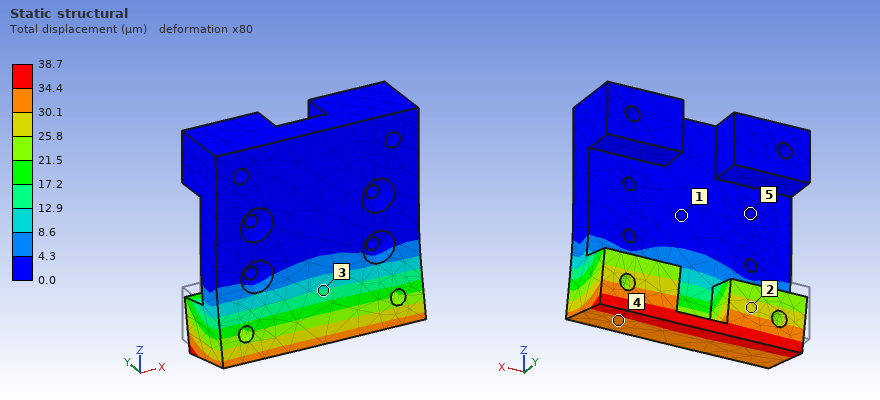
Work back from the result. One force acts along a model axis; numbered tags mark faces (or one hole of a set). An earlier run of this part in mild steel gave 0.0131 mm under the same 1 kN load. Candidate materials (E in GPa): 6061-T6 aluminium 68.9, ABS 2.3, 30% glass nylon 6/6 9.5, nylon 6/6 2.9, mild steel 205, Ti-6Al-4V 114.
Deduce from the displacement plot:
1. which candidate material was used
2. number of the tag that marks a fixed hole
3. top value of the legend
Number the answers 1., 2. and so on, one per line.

1. 6061-T6 aluminium
2. 5
3. 38.7 µm
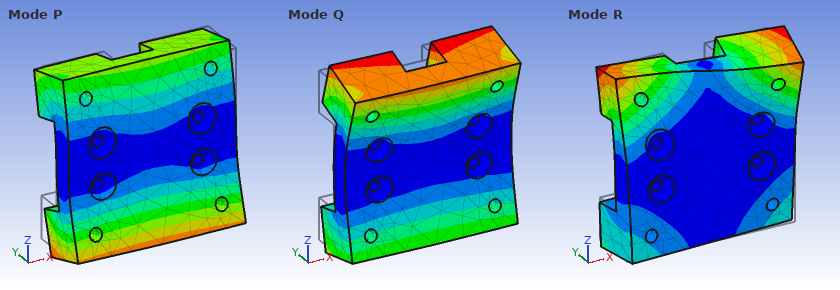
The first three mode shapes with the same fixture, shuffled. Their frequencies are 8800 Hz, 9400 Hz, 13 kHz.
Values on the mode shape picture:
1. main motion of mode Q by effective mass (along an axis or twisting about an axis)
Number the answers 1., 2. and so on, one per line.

1. along Y
